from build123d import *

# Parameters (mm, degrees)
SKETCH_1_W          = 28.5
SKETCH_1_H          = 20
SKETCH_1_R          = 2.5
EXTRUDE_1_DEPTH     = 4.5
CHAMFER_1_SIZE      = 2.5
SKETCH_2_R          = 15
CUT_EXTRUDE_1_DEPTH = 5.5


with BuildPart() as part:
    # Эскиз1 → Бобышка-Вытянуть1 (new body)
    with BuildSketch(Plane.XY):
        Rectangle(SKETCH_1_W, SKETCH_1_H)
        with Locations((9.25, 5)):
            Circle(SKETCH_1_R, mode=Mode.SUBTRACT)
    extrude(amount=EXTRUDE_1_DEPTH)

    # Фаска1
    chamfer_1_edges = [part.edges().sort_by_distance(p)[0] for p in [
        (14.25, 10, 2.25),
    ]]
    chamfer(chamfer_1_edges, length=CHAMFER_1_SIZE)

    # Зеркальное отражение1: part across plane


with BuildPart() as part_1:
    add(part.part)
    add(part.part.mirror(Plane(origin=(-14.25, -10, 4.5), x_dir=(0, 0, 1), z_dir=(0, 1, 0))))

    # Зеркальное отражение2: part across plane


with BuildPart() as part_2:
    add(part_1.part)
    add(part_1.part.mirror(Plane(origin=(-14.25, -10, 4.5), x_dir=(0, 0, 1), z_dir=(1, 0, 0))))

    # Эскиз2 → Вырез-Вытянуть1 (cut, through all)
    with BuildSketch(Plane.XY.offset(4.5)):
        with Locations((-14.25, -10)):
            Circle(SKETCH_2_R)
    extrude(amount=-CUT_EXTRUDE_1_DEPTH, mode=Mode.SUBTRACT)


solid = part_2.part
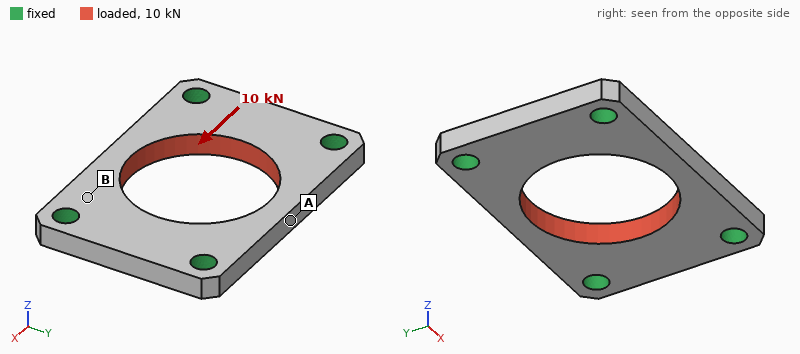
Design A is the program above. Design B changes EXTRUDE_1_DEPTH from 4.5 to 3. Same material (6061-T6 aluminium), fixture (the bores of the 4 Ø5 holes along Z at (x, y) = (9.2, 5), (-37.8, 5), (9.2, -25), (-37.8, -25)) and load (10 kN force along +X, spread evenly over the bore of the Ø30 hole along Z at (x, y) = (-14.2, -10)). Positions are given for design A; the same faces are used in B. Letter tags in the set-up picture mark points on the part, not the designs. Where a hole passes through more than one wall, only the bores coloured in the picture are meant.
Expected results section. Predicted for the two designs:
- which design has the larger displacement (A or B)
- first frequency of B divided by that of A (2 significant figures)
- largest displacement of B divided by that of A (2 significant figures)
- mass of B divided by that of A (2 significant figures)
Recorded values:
B
0.71
1.5
0.67
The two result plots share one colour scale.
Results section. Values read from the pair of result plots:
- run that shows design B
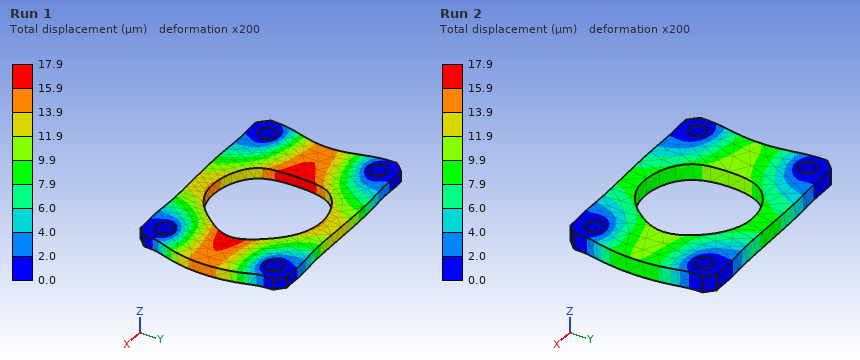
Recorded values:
Run 1
